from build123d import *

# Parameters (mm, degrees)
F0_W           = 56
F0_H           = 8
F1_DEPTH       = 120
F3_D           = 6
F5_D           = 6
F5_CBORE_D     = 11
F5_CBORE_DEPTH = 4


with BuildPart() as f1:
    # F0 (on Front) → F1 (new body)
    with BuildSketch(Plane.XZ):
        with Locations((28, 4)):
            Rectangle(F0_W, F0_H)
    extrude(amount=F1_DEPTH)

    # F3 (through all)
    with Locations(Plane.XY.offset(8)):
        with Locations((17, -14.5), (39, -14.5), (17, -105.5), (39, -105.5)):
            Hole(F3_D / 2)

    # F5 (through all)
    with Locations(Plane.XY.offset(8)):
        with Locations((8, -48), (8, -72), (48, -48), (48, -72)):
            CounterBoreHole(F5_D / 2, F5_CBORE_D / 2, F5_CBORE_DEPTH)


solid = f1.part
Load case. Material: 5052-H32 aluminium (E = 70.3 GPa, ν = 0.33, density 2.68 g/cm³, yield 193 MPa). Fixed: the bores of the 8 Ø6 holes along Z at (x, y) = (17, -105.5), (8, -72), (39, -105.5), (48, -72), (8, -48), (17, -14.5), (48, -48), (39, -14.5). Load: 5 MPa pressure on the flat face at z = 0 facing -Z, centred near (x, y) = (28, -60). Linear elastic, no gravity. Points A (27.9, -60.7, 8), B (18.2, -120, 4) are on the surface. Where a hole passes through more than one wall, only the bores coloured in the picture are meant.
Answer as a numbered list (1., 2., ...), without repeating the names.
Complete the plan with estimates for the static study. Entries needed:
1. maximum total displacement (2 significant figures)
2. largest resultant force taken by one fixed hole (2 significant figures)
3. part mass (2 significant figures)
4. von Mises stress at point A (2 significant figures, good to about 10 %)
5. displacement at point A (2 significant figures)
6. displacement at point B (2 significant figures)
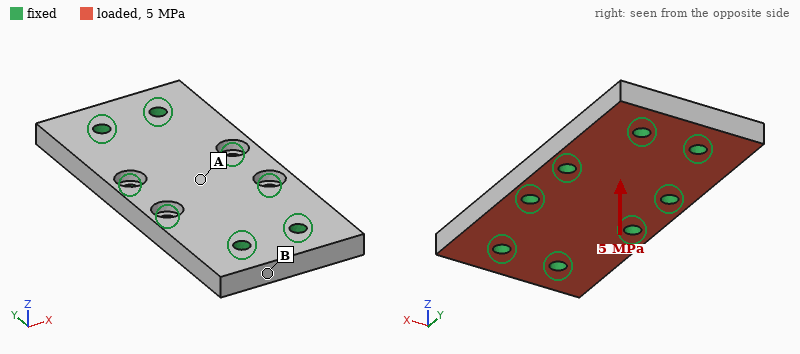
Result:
1. 25 µm
2. 4.5 kN
3. 140 g
4. 37 MPa
5. 23 µm
6. 7.8 µm
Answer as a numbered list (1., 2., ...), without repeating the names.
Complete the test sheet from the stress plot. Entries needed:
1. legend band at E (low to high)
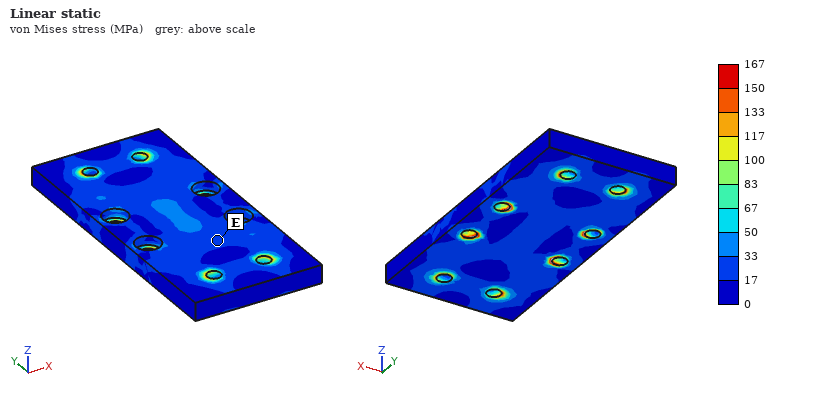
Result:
1. 17 to 33 MPa
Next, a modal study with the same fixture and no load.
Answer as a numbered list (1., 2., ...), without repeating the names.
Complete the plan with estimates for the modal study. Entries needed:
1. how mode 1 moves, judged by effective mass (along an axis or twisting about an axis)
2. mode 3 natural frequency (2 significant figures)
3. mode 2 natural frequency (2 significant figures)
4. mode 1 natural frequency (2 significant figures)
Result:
1. along Z
2. 20 kHz
3. 20 kHz
4. 18 kHz
